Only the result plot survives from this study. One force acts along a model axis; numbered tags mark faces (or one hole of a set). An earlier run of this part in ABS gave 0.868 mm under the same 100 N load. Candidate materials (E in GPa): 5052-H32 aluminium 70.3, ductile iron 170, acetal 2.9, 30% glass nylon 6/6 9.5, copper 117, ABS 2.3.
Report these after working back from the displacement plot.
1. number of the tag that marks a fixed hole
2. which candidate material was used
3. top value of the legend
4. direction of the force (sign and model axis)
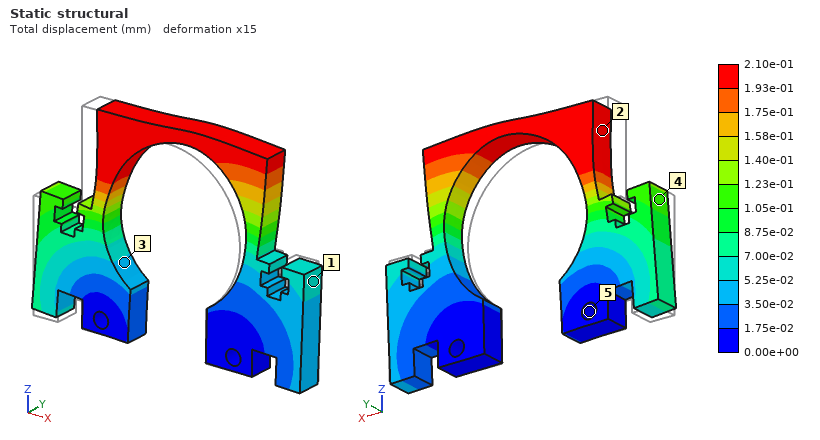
5
30% glass nylon 6/6
2.10e-01 mm
+X
